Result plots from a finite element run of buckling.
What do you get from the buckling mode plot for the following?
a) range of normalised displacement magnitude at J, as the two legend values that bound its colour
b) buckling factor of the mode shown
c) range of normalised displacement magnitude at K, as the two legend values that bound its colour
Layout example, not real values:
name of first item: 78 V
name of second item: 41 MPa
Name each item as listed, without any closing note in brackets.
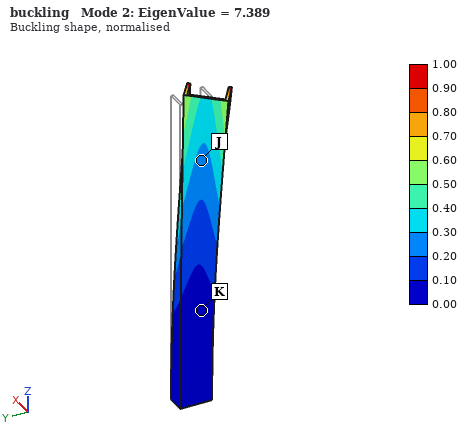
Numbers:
range of normalised displacement magnitude at J, as the two legend values that bound its colour: 0.20 to 0.30
buckling factor of the mode shown: 7.389
range of normalised displacement magnitude at K, as the two legend values that bound its colour: 0.00 to 0.10
